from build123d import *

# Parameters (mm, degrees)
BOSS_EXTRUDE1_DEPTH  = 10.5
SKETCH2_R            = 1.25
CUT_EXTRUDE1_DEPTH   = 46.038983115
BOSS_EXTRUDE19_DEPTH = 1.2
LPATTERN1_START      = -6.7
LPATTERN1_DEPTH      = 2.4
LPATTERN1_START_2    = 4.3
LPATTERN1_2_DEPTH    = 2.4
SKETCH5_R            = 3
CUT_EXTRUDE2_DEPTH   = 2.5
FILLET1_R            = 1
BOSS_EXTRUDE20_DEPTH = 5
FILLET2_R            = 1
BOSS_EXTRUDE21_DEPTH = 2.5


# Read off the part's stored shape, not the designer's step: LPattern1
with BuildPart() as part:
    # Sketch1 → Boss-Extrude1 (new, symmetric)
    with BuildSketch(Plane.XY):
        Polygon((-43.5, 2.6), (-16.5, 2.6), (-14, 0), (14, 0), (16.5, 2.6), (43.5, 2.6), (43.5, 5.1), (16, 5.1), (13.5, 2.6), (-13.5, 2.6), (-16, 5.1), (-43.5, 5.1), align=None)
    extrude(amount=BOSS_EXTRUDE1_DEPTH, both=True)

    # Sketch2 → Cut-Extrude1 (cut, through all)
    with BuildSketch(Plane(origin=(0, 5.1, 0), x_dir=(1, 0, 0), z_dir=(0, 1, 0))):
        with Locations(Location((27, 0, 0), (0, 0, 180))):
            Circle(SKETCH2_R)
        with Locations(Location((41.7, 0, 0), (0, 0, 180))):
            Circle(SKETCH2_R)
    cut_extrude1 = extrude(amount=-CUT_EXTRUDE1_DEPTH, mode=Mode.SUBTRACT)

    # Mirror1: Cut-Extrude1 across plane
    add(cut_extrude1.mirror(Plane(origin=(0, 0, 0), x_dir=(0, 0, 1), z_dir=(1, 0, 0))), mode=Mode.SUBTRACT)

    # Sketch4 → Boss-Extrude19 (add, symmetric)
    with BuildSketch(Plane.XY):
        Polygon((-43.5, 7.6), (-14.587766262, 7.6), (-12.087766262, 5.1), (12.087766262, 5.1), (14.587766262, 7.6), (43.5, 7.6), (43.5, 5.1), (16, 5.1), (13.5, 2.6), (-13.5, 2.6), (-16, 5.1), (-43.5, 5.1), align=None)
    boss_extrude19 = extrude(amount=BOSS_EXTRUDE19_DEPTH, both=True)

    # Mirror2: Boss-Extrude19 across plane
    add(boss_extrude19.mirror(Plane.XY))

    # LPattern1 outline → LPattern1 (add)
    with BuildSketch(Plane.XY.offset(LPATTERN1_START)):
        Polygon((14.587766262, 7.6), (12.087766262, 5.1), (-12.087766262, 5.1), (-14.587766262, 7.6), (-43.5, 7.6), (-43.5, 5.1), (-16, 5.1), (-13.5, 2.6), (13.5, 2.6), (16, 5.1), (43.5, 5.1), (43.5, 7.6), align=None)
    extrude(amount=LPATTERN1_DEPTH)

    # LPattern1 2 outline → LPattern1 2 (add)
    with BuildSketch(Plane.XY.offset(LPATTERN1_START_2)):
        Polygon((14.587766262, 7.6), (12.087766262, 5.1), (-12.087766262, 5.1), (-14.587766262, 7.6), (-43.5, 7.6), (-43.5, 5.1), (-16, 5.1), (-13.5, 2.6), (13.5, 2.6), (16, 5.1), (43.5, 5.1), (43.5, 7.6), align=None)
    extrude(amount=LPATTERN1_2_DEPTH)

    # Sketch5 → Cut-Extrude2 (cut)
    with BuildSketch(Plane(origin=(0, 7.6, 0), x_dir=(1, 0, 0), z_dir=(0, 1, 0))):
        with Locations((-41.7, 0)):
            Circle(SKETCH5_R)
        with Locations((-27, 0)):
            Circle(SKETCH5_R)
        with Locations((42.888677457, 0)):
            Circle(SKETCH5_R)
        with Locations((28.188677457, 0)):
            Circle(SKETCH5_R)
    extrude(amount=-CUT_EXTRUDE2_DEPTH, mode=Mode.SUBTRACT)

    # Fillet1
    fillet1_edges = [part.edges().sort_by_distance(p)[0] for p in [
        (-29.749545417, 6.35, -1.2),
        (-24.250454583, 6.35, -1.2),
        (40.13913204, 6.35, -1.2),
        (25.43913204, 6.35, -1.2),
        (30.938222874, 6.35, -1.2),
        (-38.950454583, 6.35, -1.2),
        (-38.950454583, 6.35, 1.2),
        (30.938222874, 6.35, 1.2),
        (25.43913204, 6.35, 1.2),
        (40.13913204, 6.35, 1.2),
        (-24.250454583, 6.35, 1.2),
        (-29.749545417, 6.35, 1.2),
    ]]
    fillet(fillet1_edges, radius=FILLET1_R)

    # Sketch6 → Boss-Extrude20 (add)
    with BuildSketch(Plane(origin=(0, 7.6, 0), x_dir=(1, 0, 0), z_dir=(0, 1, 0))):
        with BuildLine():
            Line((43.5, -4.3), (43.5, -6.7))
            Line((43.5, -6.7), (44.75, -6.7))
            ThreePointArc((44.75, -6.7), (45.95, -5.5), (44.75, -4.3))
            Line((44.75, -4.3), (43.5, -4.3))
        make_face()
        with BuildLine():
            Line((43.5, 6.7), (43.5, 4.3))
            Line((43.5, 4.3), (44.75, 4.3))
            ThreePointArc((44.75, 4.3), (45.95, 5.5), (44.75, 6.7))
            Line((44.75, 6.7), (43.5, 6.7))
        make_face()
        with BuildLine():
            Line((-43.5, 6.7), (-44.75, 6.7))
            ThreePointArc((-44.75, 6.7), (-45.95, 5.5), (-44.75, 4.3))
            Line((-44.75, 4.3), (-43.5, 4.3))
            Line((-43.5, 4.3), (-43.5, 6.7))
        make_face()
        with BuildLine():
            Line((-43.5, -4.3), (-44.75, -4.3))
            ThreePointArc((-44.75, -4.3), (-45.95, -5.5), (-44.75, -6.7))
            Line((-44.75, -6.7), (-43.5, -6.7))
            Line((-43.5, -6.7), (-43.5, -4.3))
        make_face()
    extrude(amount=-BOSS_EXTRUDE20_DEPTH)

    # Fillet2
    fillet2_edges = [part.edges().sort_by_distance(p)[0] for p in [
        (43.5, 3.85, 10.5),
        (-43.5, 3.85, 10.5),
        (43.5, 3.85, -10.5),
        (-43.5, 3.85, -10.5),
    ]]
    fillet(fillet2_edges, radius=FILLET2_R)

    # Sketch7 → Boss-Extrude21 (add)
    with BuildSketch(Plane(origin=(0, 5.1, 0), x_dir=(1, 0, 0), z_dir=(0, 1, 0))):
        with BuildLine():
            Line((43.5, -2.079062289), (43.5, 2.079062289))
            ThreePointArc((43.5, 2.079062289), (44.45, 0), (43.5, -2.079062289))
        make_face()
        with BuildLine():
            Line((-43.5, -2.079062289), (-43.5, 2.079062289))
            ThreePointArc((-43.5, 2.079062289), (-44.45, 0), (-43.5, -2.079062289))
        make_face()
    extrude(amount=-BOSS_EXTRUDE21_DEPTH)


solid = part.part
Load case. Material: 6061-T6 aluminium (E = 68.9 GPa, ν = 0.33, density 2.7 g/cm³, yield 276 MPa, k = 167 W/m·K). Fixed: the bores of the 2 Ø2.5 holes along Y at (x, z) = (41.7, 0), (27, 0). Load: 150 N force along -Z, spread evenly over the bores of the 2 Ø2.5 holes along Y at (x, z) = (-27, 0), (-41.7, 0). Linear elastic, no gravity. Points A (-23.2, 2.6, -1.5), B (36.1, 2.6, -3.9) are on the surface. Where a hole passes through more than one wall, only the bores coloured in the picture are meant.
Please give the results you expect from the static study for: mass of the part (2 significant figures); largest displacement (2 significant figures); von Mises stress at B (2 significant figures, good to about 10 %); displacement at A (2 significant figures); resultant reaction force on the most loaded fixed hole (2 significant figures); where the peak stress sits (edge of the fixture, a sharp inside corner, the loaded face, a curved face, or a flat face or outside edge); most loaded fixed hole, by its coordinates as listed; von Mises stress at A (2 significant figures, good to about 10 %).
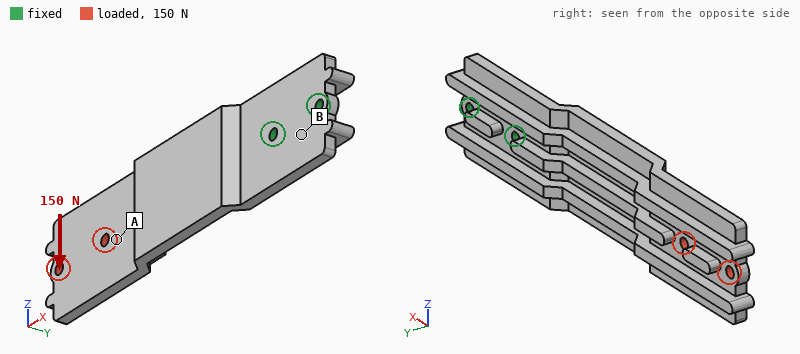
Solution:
17 g
0.24 mm
24 MPa
0.14 mm
690 N
edge of the fixture
(27, 0)
9.6 MPa
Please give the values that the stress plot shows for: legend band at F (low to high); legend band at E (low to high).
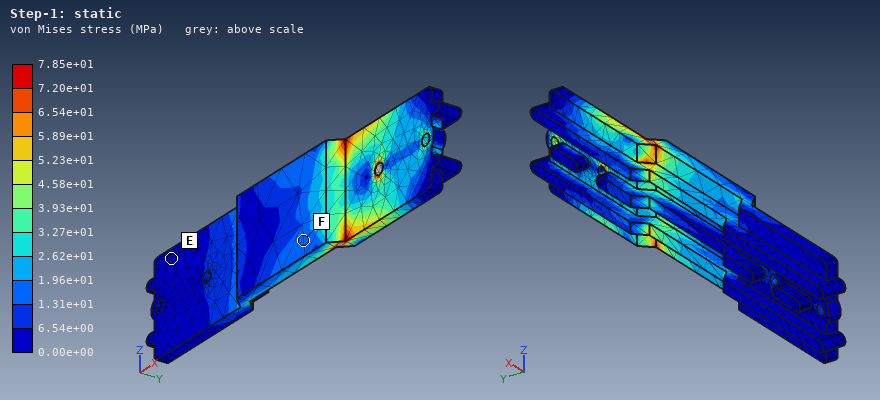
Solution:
1.31e+01 to 1.96e+01 MPa
0.00e+00 to 6.54e+00 MPa
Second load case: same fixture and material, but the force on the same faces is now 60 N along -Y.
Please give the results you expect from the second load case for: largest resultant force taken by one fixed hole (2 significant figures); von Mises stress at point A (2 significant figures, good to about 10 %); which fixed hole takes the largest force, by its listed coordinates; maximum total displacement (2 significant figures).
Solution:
250 N
13 MPa
(27, 0)
0.91 mm
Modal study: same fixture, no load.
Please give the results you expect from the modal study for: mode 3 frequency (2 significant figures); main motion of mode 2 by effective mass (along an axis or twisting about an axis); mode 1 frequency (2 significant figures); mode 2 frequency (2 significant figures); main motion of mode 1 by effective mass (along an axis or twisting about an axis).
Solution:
3000 Hz
along Z
640 Hz
1900 Hz
along Y
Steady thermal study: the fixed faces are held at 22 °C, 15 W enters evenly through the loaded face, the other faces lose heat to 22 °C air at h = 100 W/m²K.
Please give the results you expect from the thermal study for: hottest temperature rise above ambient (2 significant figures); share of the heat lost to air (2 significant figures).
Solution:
48 K
66 %
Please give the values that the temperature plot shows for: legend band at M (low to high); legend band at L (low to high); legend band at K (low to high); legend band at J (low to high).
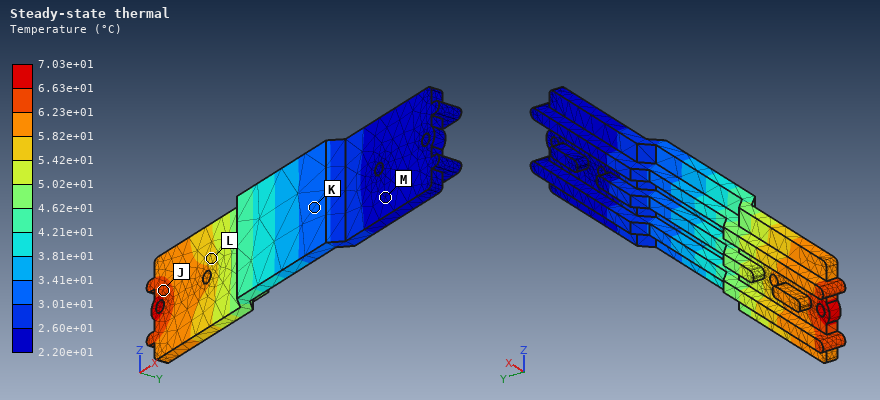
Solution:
2.20e+01 to 2.60e+01 °C
5.42e+01 to 5.82e+01 °C
3.01e+01 to 3.41e+01 °C
6.23e+01 to 6.63e+01 °C
